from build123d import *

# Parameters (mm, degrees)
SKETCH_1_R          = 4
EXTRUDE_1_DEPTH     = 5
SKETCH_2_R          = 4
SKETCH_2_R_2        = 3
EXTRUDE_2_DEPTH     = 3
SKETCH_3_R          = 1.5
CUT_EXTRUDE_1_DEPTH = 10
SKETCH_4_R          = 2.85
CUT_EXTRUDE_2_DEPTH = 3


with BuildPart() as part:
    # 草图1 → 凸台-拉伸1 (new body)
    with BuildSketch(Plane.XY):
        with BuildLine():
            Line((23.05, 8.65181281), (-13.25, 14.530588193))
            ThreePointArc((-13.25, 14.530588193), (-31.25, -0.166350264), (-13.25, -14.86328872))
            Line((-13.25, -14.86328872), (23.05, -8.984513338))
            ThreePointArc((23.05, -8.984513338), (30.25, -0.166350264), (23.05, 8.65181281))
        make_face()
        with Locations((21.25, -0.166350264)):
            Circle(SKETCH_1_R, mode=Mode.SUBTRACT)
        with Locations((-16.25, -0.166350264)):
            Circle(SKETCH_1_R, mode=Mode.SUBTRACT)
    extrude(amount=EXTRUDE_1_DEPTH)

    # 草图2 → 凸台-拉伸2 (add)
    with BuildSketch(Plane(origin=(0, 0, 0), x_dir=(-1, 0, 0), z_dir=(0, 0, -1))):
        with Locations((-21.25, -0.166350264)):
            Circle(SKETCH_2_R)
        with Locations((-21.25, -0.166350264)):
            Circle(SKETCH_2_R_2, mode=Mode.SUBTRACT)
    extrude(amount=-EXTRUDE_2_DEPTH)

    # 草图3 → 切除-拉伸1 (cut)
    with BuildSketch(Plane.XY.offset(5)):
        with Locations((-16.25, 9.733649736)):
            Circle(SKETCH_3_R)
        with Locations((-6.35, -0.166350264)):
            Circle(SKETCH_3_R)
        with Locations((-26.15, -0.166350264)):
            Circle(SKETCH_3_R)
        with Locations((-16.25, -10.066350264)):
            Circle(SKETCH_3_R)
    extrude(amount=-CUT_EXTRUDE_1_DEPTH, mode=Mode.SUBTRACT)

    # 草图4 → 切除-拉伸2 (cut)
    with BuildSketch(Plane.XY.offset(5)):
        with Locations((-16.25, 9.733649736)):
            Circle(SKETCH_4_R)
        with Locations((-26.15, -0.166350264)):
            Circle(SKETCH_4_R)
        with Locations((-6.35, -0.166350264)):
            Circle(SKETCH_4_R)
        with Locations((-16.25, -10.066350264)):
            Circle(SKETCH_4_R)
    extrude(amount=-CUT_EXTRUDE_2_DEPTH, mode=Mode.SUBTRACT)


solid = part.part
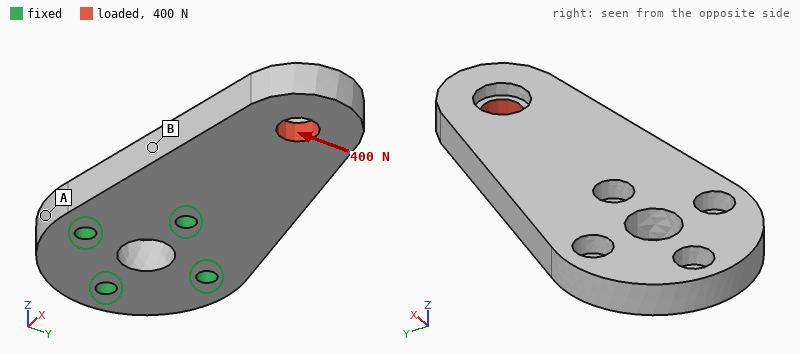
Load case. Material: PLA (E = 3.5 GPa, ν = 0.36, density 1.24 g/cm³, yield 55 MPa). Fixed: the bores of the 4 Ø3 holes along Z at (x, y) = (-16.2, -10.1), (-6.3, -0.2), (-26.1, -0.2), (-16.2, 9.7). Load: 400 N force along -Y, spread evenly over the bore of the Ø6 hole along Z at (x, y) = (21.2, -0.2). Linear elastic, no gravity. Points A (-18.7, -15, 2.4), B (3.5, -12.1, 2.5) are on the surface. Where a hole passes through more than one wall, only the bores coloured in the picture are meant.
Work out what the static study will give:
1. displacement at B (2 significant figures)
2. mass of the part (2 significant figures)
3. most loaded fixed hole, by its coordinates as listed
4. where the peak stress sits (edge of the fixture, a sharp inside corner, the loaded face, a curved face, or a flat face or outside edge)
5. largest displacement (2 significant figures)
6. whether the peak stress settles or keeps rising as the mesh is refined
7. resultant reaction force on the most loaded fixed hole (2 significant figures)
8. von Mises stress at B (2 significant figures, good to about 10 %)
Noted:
0.17 mm
7.6 g
(-6.3, -0.2)
edge of the fixture
0.53 mm
keeps rising
490 N
17 MPa
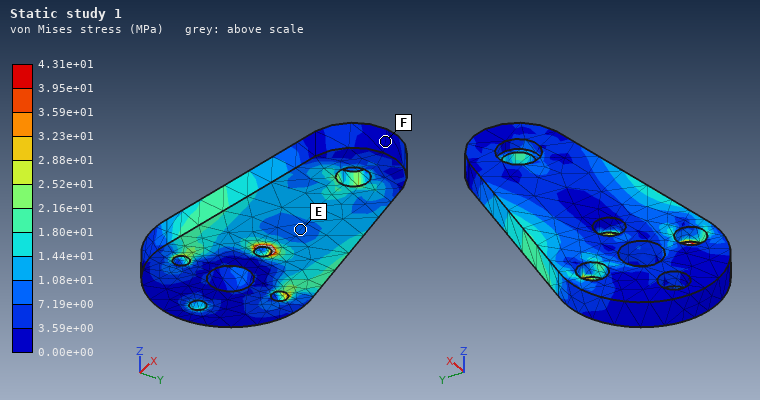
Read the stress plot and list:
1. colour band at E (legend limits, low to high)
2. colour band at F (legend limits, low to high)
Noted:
7.19e+00 to 1.08e+01 MPa
0.00e+00 to 3.59e+00 MPa
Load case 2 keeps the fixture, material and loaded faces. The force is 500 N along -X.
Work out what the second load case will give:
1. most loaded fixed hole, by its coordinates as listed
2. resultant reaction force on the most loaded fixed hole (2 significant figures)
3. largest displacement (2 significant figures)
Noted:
(-6.3, -0.2)
250 N
0.36 mm
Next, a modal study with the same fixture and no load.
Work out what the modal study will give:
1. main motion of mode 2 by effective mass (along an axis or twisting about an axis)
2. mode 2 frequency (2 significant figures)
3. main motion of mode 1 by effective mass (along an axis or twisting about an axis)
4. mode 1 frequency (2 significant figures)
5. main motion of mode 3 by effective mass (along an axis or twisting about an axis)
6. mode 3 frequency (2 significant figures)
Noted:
twisting about X
3200 Hz
along Z
1100 Hz
along Y
3700 Hz
